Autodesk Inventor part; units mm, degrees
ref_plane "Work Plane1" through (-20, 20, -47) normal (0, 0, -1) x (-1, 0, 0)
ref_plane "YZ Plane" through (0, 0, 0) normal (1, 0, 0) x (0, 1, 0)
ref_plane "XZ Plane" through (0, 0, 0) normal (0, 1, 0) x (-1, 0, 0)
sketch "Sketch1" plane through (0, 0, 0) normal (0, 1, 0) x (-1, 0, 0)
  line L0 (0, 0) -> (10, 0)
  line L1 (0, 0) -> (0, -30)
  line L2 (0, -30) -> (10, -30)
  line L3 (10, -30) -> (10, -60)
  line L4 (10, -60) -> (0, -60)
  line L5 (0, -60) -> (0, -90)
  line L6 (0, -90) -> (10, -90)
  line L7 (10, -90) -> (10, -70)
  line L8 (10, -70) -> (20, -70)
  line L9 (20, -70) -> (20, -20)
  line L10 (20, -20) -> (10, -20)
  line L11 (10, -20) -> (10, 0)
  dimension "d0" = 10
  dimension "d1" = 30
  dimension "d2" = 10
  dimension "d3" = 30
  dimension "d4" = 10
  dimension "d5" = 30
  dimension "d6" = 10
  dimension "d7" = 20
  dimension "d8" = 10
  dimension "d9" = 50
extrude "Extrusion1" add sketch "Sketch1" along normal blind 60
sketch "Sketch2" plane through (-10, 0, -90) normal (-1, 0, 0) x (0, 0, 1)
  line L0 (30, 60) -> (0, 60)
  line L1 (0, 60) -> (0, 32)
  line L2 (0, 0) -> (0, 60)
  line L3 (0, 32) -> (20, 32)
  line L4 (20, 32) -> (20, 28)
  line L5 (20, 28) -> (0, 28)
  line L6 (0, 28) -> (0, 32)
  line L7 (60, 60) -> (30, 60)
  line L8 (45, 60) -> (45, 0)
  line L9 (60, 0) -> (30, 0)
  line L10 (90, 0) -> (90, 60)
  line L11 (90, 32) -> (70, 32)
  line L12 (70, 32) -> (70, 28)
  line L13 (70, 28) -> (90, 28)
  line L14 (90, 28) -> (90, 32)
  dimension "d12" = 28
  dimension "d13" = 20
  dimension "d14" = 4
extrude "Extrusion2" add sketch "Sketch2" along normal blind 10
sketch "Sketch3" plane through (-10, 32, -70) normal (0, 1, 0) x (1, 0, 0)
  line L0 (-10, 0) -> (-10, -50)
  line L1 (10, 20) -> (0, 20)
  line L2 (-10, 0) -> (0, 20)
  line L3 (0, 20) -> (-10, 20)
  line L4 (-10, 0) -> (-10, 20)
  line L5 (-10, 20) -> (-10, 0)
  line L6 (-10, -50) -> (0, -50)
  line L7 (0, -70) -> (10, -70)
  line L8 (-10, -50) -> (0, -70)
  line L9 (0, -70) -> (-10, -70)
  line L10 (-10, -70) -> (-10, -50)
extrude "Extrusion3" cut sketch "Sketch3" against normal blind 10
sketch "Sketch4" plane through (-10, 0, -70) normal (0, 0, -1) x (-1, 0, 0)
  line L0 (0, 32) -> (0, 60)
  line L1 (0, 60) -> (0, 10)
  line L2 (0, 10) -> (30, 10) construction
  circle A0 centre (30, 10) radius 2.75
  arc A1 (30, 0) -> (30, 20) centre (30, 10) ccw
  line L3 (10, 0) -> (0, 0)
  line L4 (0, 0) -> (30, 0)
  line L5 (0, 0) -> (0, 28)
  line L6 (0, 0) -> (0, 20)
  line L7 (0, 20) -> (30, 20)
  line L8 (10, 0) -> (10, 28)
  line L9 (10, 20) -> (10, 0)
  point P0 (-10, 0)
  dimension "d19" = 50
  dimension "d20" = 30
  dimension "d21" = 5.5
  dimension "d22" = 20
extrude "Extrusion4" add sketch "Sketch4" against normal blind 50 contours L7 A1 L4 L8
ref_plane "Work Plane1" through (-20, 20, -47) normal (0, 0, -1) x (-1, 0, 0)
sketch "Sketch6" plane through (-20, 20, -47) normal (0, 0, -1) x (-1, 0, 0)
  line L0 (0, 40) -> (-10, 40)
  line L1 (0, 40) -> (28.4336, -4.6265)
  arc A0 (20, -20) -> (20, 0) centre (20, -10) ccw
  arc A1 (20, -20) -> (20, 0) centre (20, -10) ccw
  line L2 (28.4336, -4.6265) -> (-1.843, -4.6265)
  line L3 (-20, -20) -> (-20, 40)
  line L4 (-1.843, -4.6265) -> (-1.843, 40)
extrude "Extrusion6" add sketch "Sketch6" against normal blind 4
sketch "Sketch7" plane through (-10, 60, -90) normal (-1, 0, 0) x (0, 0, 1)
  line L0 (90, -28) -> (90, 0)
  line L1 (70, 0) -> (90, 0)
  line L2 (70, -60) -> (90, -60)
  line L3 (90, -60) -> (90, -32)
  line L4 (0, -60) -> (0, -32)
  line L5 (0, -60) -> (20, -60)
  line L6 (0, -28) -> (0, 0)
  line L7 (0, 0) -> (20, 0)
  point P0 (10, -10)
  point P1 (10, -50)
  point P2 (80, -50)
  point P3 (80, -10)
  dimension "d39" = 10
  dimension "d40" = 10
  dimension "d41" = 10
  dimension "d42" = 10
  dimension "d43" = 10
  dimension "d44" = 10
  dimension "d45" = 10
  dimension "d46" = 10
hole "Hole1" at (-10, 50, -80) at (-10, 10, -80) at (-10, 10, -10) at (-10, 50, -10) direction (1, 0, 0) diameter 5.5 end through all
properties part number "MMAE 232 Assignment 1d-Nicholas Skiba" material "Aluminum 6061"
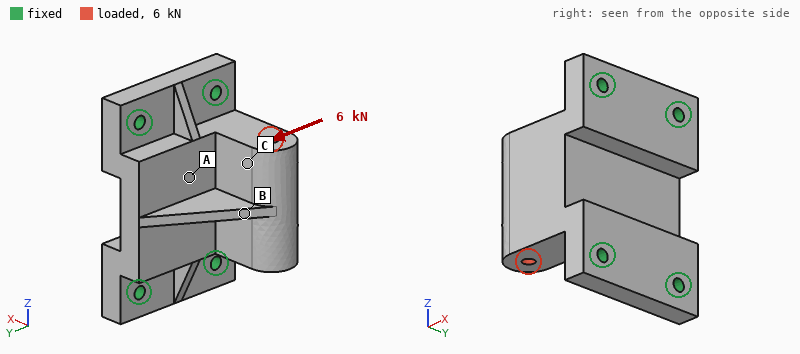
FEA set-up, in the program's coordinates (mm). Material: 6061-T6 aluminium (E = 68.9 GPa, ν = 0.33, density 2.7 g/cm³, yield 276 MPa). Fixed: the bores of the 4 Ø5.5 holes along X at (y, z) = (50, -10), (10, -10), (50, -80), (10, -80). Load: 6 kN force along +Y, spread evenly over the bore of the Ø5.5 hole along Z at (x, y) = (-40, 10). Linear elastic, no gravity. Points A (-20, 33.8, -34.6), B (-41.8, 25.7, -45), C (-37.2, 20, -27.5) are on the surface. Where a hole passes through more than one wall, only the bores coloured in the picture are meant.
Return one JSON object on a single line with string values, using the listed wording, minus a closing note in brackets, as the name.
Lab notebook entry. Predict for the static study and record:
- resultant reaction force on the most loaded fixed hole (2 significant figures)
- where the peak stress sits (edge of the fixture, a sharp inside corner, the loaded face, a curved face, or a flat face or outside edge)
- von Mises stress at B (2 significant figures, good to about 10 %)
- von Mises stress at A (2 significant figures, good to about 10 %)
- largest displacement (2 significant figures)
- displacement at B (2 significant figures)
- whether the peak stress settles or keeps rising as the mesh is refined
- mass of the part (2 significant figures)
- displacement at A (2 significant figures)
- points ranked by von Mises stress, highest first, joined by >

{"resultant reaction force on the most loaded fixed hole": "4.2 kN", "where the peak stress sits": "edge of the fixture", "von Mises stress at B": "48 MPa", "von Mises stress at A": "17 MPa", "largest displacement": "77 µm", "displacement at B": "55 µm", "whether the peak stress settles or keeps rising as the mesh is refined": "keeps rising", "mass of the part": "260 g", "displacement at A": "18 µm", "points ranked by von Mises stress, highest first, joined by >": "B > A > C"}
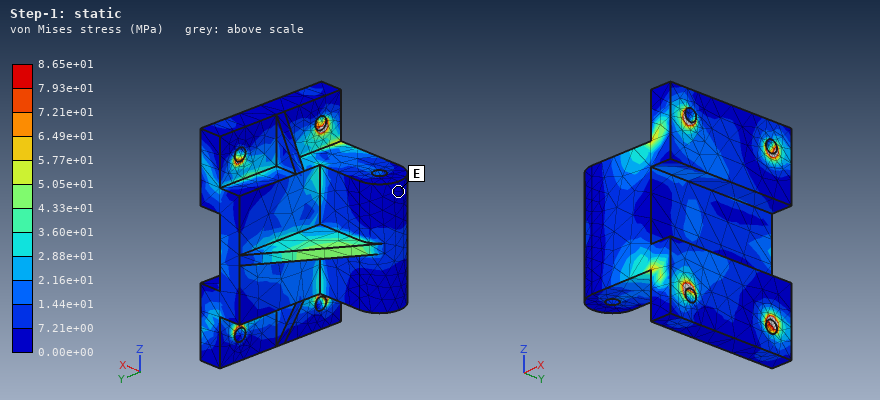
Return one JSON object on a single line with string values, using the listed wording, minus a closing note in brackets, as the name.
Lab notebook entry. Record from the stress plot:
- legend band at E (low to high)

{"legend band at E": "0.00e+00 to 7.21e+00 MPa"}
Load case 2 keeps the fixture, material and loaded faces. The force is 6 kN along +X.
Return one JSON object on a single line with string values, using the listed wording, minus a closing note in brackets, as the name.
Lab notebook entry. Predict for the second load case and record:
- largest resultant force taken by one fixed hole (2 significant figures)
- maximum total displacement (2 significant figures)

{"largest resultant force taken by one fixed hole": "3.5 kN", "maximum total displacement": "27 µm"}
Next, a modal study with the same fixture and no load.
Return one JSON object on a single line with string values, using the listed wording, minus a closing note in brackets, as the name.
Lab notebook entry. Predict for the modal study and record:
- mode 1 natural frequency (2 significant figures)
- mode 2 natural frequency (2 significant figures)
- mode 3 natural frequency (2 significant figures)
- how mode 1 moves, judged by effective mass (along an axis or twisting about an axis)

{"mode 1 natural frequency": "6000 Hz", "mode 2 natural frequency": "9000 Hz", "mode 3 natural frequency": "9100 Hz", "how mode 1 moves, judged by effective mass": "along Y"}
